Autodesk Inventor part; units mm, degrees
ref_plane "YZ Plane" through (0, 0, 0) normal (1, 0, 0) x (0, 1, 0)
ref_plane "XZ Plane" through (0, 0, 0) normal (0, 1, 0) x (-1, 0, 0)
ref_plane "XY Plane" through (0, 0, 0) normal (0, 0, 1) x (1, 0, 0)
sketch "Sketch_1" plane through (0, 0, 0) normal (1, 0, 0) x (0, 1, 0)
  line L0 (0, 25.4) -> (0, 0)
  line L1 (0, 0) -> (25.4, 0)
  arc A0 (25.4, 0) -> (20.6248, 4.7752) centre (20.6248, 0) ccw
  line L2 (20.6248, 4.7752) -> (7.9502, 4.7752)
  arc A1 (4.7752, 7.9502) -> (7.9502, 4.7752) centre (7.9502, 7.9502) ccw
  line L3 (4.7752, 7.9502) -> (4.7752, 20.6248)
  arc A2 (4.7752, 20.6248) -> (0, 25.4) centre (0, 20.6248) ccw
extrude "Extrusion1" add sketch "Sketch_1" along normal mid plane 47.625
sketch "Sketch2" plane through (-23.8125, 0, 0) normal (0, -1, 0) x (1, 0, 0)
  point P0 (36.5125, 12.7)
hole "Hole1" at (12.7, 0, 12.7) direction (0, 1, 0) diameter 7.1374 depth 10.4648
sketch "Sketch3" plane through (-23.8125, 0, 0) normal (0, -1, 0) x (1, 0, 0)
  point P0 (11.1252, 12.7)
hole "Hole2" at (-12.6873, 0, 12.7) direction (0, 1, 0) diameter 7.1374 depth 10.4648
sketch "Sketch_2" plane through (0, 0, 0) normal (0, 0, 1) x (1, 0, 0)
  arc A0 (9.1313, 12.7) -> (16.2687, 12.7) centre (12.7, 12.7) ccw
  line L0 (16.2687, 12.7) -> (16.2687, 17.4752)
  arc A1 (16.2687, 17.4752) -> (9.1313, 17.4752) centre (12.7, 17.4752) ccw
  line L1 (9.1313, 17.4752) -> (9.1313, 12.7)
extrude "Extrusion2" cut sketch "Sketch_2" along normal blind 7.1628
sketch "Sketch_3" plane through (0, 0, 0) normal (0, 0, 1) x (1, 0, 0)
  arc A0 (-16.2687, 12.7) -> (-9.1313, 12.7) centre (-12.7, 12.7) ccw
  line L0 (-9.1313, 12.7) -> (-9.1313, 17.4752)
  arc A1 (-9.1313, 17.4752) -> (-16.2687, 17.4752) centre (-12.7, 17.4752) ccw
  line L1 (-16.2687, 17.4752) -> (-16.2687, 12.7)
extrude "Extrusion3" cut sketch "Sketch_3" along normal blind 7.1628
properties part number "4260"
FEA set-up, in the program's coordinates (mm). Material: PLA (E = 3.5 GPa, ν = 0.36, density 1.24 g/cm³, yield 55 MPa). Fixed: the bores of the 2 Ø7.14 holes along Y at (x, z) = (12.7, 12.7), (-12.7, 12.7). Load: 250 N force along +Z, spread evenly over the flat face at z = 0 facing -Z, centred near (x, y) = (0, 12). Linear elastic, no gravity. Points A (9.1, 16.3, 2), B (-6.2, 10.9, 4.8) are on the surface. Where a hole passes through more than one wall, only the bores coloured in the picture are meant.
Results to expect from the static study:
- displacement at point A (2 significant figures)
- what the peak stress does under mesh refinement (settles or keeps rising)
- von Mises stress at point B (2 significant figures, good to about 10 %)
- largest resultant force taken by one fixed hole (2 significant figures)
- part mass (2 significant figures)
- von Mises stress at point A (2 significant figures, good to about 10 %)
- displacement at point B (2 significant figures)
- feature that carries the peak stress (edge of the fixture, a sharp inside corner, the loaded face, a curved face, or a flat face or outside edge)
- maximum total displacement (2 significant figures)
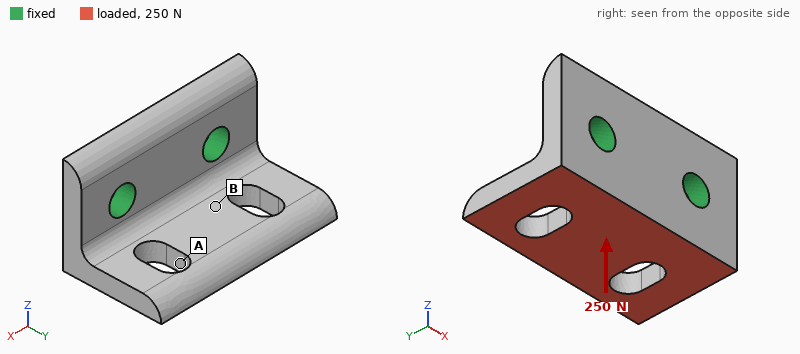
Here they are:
0.22 mm
keeps rising
7.4 MPa
130 N
11 g
2.8 MPa
0.11 mm
edge of the fixture
0.43 mm
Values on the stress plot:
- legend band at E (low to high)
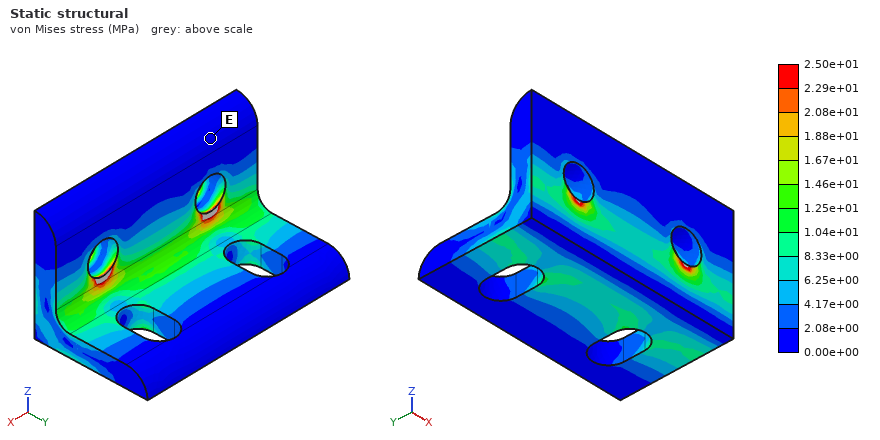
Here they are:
0.00e+00 to 2.08e+00 MPa
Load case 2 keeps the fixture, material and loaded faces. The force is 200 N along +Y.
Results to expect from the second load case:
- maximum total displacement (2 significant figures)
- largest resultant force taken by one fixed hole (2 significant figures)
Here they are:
0.21 mm
100 N
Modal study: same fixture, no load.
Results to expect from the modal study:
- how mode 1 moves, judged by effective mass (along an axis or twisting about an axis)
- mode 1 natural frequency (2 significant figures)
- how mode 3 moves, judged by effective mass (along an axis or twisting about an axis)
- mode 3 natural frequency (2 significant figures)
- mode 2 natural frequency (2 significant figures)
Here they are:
along Z
2000 Hz
along X
4800 Hz
2900 Hz
